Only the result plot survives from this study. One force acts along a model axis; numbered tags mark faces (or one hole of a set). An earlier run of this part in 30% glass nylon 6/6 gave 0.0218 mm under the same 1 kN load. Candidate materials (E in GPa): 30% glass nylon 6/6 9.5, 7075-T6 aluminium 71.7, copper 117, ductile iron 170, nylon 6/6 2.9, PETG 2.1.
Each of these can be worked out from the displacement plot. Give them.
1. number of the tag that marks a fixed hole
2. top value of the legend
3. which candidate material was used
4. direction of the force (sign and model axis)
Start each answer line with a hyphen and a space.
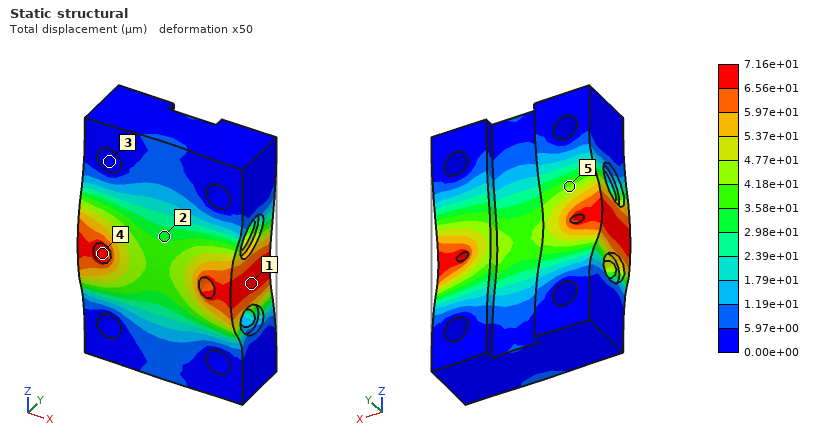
- 3
- 7.16e+01 µm
- nylon 6/6
- -Y
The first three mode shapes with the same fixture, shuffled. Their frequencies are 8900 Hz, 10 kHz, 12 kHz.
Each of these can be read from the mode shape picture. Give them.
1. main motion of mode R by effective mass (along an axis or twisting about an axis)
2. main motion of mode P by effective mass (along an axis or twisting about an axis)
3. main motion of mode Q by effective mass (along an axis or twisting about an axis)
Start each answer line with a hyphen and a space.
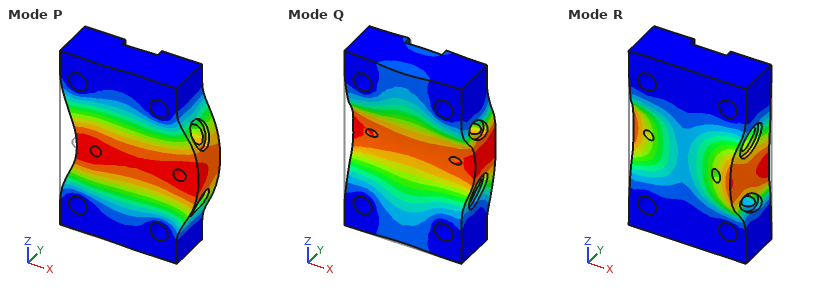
- twisting about Z
- along X
- along Y
